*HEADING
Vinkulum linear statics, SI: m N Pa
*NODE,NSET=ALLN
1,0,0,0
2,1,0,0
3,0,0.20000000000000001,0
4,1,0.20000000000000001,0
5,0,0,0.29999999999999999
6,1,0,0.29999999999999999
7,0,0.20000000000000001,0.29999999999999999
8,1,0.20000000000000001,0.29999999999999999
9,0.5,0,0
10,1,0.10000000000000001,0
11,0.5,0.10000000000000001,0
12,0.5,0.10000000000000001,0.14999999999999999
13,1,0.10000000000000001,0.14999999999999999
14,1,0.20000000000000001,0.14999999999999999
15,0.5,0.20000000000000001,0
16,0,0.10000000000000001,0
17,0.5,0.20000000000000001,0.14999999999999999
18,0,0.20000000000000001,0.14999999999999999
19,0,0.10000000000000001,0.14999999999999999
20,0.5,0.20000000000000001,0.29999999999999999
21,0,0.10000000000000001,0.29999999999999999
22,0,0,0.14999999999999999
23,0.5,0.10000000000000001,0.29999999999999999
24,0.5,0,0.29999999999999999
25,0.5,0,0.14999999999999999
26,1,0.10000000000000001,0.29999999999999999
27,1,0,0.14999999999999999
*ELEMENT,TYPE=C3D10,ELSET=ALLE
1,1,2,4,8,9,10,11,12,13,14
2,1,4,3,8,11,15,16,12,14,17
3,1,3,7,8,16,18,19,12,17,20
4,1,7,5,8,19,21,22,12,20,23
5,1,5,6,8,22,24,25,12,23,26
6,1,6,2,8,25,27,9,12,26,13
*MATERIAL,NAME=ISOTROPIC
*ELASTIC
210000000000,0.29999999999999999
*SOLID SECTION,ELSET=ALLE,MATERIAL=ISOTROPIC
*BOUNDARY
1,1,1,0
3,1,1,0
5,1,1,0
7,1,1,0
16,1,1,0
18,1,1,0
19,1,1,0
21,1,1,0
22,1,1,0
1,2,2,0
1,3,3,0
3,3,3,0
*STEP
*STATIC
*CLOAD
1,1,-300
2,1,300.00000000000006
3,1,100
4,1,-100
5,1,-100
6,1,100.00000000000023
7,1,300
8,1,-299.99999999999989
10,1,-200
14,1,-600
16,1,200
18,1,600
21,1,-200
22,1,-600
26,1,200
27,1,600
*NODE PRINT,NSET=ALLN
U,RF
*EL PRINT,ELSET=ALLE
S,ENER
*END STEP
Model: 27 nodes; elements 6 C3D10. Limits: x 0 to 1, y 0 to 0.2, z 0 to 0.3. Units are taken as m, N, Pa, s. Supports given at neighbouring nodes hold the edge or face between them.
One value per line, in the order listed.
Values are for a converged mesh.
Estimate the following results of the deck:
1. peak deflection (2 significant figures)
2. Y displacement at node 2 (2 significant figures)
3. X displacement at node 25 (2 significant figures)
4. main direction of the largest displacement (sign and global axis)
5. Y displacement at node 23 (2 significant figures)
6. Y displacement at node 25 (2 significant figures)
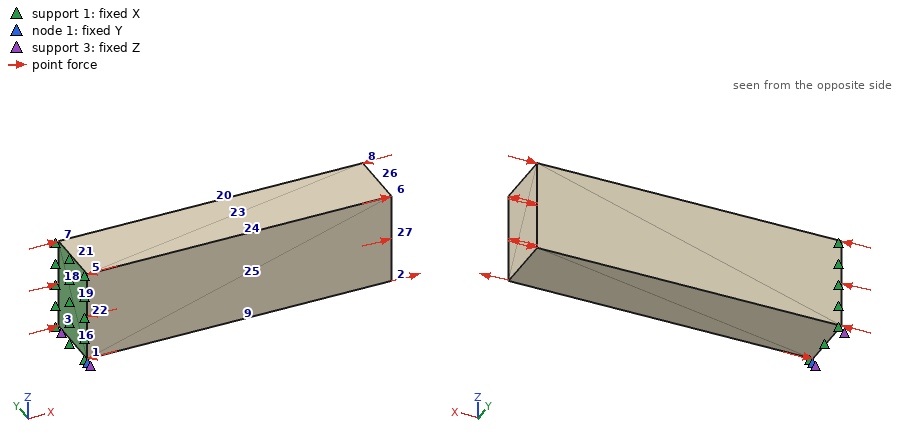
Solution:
2.5e-06 m
2.4e-06 m
2.4e-07 m
+Y
5.3e-07 m
5.8e-07 m
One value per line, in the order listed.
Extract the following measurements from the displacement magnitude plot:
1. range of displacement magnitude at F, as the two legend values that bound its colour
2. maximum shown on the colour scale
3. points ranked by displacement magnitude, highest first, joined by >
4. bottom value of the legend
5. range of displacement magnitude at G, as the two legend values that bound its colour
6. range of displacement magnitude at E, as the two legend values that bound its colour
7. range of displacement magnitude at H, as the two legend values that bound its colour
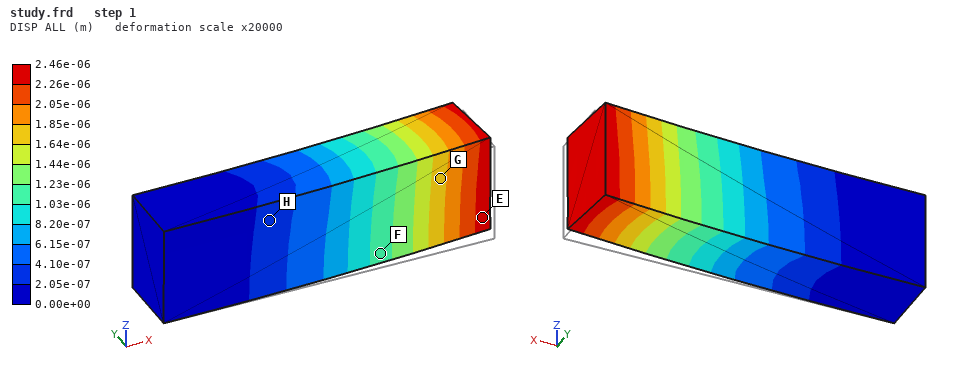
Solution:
1.03e-06 to 1.23e-06 m
2.46e-06 m
E > G > F > H
0.00e+00 m
1.64e-06 to 1.85e-06 m
2.26e-06 to 2.46e-06 m
2.05e-07 to 4.10e-07 m
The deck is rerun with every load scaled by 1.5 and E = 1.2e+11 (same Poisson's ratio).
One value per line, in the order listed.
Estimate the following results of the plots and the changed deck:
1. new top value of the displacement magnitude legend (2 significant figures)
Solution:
6.5e-06 m
